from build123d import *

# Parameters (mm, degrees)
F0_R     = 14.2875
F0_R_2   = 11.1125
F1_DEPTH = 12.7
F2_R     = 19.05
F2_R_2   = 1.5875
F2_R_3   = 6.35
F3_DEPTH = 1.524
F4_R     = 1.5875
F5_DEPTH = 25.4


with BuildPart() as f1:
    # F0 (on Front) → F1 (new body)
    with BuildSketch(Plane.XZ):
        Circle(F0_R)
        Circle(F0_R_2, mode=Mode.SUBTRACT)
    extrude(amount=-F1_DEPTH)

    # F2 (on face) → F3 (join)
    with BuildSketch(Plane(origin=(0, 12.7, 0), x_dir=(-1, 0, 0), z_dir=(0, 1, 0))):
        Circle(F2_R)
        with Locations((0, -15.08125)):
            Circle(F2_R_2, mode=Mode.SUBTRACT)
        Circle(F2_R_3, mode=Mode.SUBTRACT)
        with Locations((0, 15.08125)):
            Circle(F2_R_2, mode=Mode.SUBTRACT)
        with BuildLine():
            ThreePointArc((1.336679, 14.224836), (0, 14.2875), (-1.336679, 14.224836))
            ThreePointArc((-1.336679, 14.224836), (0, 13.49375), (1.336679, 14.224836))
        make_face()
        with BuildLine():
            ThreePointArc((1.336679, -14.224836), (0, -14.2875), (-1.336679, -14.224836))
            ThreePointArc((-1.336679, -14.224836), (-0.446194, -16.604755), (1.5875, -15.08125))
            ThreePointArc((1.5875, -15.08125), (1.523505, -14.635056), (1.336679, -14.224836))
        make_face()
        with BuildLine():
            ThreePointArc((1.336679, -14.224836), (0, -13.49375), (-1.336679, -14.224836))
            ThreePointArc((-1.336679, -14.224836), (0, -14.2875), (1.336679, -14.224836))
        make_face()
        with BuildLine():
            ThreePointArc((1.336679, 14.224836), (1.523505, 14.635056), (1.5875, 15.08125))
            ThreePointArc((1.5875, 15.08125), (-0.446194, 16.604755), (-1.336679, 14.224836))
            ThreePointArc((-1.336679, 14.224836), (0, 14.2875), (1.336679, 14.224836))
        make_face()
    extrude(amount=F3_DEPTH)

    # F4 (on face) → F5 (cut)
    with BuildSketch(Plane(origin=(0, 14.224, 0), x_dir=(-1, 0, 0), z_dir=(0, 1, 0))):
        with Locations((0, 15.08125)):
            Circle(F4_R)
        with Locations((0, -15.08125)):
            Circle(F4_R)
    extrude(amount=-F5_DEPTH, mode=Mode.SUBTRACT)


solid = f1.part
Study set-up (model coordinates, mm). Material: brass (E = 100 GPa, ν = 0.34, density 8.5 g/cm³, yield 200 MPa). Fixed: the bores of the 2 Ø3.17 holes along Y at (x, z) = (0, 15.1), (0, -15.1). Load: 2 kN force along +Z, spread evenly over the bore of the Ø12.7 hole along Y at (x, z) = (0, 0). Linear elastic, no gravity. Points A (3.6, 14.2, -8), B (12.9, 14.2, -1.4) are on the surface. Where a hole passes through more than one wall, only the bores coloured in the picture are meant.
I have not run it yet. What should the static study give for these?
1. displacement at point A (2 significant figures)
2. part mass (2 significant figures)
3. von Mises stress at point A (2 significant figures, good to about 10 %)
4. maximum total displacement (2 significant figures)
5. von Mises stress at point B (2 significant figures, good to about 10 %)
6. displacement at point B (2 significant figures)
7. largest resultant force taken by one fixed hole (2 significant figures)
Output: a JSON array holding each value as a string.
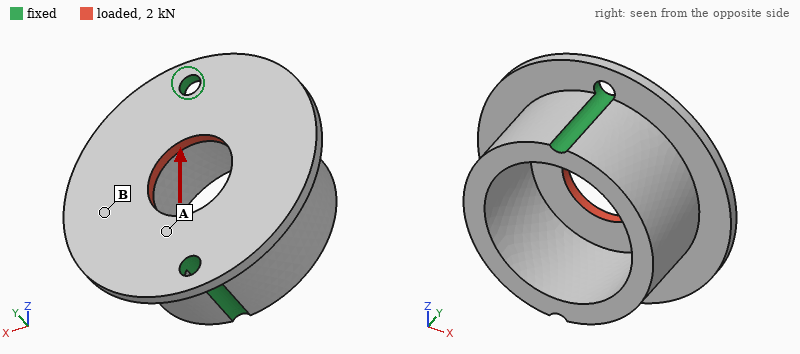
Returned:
["3.9 µm", "40 g", "45 MPa", "6.3 µm", "10 MPa", "3.2 µm", "1.0 kN"]
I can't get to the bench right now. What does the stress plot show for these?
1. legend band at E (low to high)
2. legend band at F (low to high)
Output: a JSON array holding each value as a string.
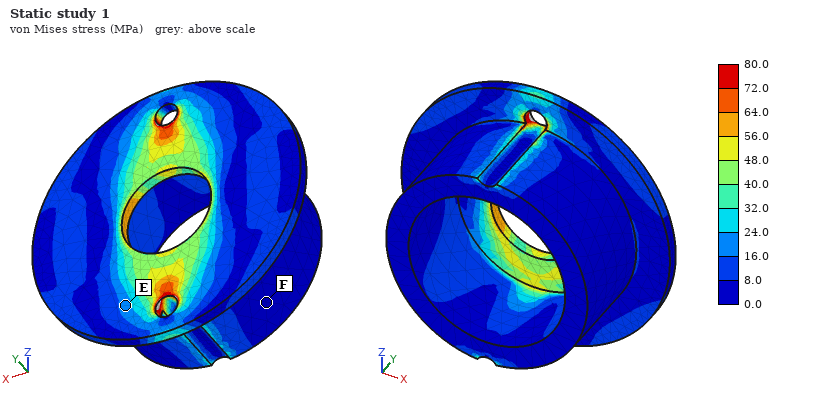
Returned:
["16.0 to 24.0 MPa", "0.0 to 8.0 MPa"]
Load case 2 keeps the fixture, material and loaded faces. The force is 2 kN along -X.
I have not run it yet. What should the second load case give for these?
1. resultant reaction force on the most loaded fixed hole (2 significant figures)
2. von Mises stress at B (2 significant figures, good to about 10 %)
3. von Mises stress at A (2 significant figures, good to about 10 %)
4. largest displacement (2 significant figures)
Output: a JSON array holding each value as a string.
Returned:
["1.0 kN", "26 MPa", "34 MPa", "9.4 µm"]
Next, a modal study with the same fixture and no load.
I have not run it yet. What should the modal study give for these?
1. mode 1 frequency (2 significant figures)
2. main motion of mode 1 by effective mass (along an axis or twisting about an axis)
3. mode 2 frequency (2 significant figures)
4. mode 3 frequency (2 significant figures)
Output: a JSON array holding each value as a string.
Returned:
["14 kHz", "twisting about Z", "15 kHz", "15 kHz"]
